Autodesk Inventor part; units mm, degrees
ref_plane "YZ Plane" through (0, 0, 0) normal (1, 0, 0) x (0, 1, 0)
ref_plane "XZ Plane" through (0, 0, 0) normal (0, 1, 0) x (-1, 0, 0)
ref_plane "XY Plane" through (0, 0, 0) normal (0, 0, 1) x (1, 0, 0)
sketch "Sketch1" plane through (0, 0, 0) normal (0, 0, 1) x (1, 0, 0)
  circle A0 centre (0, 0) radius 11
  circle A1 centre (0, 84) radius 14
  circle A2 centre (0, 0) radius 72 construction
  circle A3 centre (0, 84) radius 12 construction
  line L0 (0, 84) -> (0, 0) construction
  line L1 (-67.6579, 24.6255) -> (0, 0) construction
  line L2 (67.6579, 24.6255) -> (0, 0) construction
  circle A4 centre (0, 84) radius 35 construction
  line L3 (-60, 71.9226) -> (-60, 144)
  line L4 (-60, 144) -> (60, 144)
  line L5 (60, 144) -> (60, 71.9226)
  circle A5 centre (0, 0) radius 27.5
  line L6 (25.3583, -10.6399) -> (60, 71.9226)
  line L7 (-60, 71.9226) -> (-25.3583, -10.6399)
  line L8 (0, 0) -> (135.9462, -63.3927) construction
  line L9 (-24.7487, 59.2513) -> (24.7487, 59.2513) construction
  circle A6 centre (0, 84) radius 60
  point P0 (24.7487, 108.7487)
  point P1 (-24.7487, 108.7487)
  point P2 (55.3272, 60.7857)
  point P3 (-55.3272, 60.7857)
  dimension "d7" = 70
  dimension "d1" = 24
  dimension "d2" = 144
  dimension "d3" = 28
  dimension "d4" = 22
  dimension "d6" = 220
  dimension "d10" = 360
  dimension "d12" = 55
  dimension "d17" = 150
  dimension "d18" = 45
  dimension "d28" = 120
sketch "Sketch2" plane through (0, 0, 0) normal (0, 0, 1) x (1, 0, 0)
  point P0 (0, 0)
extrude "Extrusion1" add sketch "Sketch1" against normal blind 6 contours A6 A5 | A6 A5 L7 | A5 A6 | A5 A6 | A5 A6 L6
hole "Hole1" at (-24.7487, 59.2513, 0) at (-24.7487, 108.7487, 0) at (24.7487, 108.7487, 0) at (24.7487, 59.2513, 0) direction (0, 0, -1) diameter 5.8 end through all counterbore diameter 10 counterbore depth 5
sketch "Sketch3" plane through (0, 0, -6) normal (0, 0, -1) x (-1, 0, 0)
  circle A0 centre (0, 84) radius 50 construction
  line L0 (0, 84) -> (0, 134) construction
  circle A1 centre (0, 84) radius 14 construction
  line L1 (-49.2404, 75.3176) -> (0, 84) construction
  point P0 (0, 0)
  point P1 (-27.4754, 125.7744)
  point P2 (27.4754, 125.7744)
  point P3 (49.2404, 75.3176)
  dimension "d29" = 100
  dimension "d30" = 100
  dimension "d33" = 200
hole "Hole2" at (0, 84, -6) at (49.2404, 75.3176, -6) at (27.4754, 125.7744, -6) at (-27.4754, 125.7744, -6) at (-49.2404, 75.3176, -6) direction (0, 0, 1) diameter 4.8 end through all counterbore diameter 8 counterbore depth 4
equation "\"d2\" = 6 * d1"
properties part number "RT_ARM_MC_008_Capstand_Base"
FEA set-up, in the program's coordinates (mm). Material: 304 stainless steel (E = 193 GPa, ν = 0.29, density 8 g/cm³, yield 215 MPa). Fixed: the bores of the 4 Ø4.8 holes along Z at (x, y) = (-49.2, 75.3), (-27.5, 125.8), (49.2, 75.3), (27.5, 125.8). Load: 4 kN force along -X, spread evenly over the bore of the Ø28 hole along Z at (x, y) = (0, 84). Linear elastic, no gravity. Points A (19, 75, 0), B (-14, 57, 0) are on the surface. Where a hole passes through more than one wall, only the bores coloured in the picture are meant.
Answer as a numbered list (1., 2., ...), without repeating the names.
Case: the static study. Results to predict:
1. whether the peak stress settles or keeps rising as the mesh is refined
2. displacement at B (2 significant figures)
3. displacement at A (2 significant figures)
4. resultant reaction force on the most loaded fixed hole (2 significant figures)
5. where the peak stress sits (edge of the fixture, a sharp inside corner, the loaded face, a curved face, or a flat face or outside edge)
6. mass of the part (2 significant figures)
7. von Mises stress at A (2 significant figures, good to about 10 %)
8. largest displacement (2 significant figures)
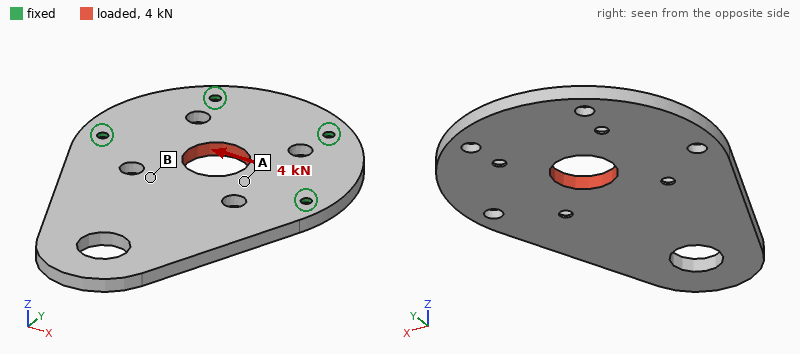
1. keeps rising
2. 2.8 µm
3. 2.9 µm
4. 1.3 kN
5. edge of the fixture
6. 640 g
7. 10 MPa
8. 3.3 µm
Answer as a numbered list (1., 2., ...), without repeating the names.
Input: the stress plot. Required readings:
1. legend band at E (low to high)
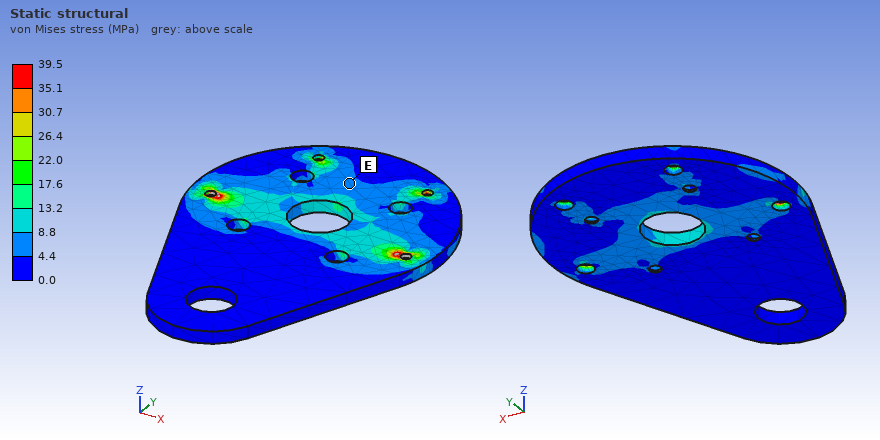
1. 4.4 to 8.8 MPa
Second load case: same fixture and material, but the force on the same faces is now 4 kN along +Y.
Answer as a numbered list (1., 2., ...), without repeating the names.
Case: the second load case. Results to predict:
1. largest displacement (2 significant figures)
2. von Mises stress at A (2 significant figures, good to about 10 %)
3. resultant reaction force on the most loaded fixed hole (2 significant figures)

1. 15 µm
2. 6.8 MPa
3. 1.0 kN
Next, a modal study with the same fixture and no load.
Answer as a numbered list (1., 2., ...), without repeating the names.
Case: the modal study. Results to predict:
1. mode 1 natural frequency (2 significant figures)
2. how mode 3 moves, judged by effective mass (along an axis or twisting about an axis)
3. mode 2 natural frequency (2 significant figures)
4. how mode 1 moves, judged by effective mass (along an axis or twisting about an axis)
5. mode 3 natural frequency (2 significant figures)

1. 490 Hz
2. along Z
3. 1900 Hz
4. along Z
5. 2100 Hz
